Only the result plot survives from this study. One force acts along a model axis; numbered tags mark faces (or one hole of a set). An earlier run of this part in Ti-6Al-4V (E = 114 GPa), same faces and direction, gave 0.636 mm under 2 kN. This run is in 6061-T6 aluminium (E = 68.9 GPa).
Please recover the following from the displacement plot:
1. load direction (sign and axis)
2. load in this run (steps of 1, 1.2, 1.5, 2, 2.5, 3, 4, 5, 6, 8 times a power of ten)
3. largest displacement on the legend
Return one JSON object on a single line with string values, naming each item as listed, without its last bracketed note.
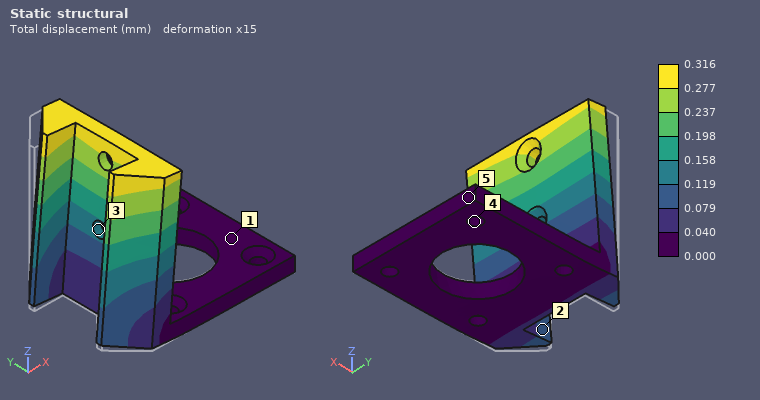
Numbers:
{"load direction": "+X", "load in this run": "600 N", "largest displacement on the legend": "0.316 mm"}
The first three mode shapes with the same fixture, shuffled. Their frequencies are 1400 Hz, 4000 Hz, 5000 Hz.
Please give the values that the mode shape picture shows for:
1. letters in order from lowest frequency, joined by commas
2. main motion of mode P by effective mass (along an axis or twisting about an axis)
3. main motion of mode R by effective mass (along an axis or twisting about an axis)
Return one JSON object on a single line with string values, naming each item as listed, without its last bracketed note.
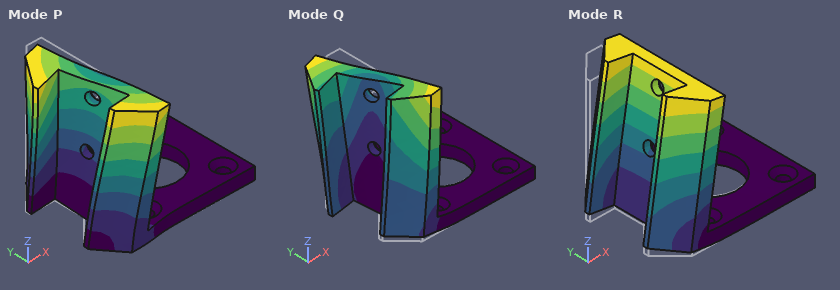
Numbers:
{"letters in order from lowest frequency, joined by commas": "R, Q, P", "main motion of mode P by effective mass": "along Y", "main motion of mode R by effective mass": "along X"}
